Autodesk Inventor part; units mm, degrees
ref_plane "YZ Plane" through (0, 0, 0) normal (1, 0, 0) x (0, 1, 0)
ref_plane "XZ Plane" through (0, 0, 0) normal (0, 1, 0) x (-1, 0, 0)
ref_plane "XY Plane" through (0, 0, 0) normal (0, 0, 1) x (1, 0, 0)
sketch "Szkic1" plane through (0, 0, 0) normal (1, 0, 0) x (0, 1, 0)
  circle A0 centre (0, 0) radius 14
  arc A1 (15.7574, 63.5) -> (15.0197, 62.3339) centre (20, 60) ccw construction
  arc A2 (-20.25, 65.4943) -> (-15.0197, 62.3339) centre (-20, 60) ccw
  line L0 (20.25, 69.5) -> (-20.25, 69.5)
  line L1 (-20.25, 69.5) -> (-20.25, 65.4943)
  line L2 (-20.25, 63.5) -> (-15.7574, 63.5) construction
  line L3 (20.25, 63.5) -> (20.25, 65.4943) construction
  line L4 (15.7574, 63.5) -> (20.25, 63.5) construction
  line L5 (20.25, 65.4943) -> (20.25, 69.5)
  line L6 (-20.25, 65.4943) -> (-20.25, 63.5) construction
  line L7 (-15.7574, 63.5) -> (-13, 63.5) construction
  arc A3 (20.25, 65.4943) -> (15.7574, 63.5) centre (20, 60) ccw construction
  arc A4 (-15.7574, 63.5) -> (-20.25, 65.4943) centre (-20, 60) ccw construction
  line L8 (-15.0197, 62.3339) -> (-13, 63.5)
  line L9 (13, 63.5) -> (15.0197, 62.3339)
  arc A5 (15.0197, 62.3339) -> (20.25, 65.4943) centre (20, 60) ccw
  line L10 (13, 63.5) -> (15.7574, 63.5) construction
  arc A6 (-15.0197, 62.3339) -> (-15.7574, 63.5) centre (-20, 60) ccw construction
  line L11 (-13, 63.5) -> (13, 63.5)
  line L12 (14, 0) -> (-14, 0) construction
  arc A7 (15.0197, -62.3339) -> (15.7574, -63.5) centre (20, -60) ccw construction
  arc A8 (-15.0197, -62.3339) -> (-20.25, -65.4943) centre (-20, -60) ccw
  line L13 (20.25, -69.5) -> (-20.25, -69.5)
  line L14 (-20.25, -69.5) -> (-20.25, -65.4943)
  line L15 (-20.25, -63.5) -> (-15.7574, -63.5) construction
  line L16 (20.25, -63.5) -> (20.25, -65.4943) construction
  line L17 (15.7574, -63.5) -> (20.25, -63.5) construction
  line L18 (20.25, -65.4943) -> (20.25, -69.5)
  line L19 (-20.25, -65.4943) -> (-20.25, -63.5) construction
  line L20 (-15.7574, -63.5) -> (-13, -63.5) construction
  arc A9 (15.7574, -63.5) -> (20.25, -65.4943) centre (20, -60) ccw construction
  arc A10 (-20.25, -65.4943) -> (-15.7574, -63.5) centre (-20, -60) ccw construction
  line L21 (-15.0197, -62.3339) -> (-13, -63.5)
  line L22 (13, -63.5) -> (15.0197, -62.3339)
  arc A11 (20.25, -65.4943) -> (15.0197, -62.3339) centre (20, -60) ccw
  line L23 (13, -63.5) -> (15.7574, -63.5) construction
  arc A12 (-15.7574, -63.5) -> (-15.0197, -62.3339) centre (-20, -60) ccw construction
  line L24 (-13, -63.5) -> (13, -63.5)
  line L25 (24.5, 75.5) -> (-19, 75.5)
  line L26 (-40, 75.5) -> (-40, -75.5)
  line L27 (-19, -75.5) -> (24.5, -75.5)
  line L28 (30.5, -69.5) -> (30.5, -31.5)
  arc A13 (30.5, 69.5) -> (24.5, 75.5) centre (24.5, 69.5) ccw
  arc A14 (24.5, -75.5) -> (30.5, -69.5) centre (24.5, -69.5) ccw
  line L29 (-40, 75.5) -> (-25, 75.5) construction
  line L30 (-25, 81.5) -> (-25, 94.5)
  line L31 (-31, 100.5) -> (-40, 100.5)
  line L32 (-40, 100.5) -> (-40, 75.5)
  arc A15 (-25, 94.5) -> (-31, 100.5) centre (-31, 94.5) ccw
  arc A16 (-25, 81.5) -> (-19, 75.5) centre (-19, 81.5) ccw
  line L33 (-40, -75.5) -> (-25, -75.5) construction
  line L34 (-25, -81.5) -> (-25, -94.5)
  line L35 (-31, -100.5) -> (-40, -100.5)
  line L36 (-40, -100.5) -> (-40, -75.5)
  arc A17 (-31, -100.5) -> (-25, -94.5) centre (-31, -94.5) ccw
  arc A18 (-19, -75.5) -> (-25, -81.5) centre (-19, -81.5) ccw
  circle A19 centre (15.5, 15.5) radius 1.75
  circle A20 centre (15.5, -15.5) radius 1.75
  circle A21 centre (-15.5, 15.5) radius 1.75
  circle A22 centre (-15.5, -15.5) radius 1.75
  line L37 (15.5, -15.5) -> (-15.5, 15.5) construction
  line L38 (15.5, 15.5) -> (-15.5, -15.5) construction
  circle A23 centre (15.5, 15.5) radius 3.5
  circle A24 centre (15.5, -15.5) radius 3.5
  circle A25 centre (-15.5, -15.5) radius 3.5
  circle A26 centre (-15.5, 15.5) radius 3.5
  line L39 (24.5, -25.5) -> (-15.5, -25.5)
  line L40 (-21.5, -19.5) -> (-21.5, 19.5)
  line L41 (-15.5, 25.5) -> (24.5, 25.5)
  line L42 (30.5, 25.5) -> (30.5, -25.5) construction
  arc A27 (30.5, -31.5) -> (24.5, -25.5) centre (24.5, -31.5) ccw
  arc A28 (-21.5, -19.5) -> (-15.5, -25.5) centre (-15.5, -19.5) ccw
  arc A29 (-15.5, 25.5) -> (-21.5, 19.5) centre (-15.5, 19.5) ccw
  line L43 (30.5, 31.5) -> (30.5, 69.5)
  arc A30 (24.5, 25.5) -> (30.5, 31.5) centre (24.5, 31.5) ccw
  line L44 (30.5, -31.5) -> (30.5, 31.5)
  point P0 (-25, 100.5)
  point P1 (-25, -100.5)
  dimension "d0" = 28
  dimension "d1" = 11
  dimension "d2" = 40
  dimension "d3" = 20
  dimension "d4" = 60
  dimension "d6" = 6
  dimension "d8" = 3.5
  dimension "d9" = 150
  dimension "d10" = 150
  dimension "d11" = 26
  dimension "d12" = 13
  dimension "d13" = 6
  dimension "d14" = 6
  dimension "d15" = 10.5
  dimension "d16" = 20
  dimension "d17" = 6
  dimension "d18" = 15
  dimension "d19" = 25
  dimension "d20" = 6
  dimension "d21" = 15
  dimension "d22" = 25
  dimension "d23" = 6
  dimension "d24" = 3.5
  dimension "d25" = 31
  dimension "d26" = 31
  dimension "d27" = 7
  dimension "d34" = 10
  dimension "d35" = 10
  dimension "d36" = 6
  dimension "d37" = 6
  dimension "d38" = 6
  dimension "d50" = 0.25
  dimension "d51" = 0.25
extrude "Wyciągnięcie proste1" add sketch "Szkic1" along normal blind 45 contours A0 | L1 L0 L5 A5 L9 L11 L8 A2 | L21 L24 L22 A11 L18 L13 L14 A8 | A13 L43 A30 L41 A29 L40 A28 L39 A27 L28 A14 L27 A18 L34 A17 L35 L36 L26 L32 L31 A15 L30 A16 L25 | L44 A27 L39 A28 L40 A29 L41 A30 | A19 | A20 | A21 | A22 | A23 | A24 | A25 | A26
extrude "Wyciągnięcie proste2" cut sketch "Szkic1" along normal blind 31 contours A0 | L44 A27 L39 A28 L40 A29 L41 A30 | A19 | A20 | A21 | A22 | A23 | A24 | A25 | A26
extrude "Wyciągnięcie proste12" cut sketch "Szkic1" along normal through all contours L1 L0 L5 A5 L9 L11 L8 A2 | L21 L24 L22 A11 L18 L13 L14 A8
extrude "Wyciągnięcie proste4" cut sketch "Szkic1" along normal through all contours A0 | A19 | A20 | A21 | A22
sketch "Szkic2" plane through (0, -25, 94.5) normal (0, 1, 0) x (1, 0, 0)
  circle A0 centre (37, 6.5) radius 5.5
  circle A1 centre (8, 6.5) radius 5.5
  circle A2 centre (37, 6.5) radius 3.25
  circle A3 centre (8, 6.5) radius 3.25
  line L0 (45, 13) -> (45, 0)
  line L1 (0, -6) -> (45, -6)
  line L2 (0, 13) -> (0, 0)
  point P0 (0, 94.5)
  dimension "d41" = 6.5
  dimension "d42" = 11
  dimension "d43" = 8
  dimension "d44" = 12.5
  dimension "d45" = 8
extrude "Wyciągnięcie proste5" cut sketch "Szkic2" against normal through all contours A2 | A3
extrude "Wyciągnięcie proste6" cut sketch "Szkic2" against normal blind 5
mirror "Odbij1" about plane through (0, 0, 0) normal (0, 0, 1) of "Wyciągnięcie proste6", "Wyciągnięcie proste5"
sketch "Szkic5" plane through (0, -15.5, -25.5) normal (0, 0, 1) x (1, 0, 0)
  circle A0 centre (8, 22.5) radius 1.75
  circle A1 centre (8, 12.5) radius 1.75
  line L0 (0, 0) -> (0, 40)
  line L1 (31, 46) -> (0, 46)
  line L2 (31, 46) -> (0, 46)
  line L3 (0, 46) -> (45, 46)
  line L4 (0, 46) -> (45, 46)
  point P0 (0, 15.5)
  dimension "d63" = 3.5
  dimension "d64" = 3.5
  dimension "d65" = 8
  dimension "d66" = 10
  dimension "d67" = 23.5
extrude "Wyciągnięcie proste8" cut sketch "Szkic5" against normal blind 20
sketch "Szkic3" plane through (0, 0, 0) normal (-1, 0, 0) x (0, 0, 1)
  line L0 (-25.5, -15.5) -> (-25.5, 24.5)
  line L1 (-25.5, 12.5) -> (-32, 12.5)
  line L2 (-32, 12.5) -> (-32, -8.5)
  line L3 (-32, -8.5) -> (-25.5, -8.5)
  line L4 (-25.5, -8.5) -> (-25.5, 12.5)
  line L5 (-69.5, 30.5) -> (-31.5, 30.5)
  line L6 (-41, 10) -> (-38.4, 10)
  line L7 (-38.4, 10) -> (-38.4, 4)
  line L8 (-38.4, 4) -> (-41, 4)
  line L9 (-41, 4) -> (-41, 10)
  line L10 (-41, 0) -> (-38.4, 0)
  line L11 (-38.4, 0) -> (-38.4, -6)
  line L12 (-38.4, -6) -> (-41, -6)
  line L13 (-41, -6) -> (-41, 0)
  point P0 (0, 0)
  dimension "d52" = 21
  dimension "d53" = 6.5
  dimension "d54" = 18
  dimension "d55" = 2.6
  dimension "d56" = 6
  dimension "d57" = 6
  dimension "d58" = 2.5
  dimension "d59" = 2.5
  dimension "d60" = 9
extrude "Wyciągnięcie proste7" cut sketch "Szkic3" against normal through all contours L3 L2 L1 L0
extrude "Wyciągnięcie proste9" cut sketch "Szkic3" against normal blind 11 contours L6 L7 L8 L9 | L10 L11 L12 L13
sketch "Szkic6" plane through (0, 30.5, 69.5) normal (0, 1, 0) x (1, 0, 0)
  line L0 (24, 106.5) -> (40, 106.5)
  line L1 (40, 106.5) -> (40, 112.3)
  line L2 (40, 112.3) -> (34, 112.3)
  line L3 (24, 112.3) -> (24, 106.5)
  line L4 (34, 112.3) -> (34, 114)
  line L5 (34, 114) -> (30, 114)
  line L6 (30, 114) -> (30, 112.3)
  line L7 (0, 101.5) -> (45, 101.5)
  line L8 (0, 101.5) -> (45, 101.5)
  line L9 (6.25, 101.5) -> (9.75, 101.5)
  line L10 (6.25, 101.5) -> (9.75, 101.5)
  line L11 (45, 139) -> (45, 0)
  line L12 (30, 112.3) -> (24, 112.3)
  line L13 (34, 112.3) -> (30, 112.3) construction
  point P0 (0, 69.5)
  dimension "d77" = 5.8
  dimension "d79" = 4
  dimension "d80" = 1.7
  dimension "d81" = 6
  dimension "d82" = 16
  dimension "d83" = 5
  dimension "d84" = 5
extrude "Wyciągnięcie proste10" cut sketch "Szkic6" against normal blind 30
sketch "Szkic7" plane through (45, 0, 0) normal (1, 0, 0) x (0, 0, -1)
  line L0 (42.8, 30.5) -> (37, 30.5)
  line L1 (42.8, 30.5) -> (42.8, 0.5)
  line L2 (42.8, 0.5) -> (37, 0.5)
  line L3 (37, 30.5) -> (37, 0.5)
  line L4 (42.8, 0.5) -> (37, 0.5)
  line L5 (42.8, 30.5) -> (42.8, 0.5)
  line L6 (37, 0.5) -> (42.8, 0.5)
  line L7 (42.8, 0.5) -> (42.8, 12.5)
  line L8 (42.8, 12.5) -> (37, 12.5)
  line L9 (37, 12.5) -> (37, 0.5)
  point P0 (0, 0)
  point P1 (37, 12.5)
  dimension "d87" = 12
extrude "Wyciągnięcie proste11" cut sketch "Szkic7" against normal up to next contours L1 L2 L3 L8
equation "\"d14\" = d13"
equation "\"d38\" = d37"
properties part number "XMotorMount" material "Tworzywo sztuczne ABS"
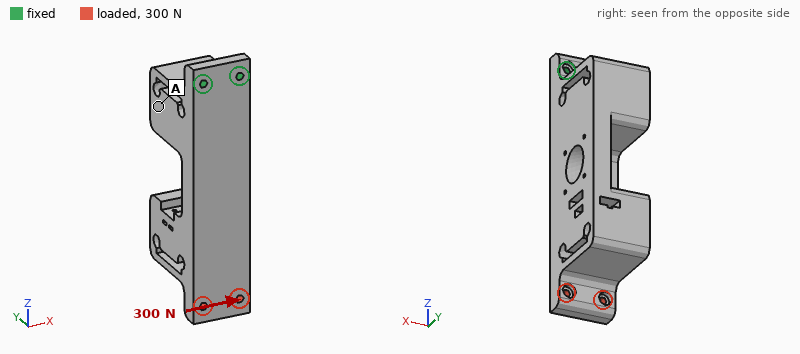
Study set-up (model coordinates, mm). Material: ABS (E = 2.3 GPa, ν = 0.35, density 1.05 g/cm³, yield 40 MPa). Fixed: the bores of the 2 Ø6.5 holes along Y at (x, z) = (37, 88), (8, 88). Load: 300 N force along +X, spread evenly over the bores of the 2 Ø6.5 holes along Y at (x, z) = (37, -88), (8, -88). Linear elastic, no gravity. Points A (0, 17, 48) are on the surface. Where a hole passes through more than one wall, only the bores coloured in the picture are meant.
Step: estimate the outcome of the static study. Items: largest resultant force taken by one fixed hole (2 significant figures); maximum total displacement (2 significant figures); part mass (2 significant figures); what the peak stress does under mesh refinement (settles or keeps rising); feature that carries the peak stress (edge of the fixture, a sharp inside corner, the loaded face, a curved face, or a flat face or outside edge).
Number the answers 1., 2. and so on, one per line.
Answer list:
1. 1.7 kN
2. 2.2 mm
3. 390 g
4. keeps rising
5. edge of the fixture
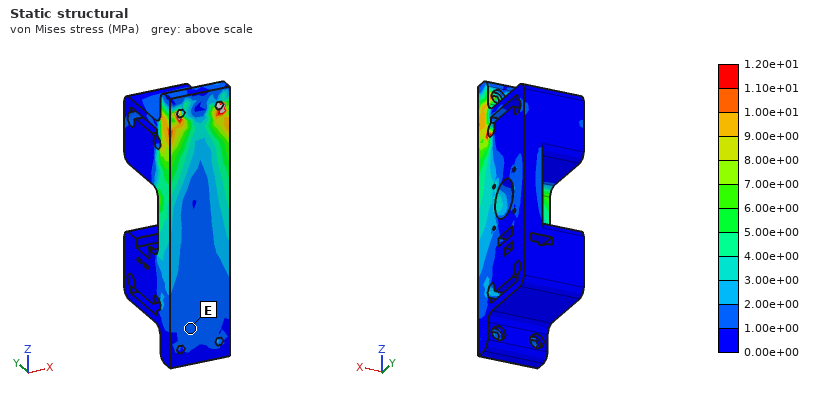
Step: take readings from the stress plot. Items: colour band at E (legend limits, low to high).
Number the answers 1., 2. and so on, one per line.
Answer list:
1. 1.00e+00 to 2.00e+00 MPa
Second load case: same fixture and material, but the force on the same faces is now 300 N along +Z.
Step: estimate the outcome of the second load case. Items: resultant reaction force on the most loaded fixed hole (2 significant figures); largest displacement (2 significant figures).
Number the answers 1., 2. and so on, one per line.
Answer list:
1. 150 N
2. 0.20 mm
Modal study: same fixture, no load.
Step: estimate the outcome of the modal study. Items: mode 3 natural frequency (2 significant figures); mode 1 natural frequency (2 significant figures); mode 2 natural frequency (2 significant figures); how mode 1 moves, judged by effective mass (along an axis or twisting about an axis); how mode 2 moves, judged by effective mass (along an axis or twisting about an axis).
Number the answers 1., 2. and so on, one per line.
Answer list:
1. 420 Hz
2. 76 Hz
3. 190 Hz
4. along Y
5. along X
